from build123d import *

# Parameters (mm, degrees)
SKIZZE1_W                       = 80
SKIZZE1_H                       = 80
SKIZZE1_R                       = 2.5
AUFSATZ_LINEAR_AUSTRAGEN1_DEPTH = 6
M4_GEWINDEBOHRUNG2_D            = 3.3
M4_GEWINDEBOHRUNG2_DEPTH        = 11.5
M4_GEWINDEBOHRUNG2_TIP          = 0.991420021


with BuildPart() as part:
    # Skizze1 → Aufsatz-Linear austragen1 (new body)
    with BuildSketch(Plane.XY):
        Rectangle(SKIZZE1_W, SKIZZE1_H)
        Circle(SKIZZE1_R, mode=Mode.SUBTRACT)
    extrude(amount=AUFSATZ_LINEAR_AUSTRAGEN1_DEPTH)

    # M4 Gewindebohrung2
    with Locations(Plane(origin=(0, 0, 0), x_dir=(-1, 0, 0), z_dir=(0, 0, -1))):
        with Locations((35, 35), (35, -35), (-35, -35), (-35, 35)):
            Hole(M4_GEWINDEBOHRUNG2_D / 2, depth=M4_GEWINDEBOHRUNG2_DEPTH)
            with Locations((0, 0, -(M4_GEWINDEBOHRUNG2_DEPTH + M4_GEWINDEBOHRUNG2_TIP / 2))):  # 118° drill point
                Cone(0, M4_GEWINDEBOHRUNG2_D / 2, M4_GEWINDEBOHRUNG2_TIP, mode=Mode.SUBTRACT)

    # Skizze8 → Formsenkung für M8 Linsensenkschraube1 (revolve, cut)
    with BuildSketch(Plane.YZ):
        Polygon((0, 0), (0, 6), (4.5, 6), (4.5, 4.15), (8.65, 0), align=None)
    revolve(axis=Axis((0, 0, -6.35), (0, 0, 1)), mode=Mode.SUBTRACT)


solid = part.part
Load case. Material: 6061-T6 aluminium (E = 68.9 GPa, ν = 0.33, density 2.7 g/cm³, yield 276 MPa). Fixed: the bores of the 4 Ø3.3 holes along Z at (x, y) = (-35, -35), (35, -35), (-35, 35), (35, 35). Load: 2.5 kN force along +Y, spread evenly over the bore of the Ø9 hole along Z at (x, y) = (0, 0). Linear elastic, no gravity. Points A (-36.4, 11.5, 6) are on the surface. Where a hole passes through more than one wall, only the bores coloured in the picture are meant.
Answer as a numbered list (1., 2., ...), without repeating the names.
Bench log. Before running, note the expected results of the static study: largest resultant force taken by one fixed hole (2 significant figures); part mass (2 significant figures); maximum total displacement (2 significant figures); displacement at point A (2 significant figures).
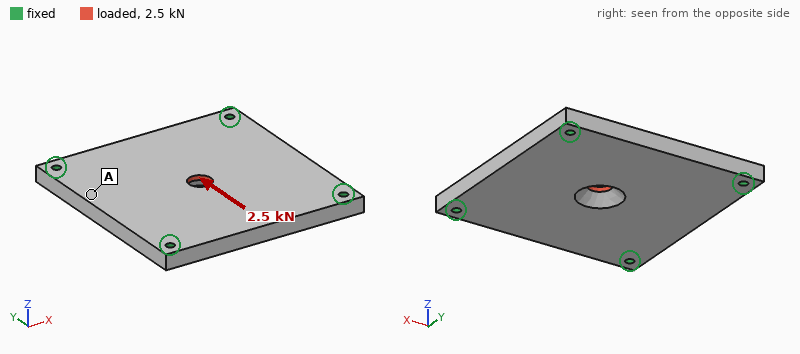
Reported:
1. 710 N
2. 100 g
3. 9.9 µm
4. 1.8 µm
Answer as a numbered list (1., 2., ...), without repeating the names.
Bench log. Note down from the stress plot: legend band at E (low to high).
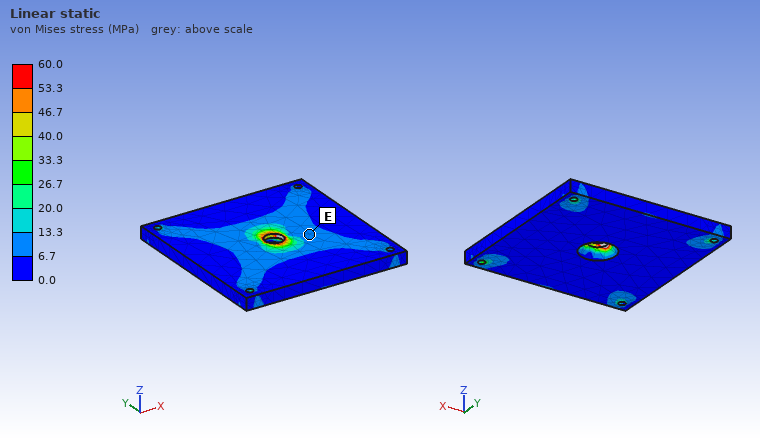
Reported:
1. 6.7 to 13.3 MPa
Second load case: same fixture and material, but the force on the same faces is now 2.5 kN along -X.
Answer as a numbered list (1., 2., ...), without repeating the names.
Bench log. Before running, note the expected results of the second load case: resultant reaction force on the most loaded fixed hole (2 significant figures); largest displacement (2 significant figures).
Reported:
1. 710 N
2. 9.9 µm
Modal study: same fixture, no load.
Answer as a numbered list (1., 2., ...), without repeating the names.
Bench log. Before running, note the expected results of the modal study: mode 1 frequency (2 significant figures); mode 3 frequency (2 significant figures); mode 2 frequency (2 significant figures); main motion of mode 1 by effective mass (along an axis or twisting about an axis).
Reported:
1. 3700 Hz
2. 6400 Hz
3. 6400 Hz
4. along Z
